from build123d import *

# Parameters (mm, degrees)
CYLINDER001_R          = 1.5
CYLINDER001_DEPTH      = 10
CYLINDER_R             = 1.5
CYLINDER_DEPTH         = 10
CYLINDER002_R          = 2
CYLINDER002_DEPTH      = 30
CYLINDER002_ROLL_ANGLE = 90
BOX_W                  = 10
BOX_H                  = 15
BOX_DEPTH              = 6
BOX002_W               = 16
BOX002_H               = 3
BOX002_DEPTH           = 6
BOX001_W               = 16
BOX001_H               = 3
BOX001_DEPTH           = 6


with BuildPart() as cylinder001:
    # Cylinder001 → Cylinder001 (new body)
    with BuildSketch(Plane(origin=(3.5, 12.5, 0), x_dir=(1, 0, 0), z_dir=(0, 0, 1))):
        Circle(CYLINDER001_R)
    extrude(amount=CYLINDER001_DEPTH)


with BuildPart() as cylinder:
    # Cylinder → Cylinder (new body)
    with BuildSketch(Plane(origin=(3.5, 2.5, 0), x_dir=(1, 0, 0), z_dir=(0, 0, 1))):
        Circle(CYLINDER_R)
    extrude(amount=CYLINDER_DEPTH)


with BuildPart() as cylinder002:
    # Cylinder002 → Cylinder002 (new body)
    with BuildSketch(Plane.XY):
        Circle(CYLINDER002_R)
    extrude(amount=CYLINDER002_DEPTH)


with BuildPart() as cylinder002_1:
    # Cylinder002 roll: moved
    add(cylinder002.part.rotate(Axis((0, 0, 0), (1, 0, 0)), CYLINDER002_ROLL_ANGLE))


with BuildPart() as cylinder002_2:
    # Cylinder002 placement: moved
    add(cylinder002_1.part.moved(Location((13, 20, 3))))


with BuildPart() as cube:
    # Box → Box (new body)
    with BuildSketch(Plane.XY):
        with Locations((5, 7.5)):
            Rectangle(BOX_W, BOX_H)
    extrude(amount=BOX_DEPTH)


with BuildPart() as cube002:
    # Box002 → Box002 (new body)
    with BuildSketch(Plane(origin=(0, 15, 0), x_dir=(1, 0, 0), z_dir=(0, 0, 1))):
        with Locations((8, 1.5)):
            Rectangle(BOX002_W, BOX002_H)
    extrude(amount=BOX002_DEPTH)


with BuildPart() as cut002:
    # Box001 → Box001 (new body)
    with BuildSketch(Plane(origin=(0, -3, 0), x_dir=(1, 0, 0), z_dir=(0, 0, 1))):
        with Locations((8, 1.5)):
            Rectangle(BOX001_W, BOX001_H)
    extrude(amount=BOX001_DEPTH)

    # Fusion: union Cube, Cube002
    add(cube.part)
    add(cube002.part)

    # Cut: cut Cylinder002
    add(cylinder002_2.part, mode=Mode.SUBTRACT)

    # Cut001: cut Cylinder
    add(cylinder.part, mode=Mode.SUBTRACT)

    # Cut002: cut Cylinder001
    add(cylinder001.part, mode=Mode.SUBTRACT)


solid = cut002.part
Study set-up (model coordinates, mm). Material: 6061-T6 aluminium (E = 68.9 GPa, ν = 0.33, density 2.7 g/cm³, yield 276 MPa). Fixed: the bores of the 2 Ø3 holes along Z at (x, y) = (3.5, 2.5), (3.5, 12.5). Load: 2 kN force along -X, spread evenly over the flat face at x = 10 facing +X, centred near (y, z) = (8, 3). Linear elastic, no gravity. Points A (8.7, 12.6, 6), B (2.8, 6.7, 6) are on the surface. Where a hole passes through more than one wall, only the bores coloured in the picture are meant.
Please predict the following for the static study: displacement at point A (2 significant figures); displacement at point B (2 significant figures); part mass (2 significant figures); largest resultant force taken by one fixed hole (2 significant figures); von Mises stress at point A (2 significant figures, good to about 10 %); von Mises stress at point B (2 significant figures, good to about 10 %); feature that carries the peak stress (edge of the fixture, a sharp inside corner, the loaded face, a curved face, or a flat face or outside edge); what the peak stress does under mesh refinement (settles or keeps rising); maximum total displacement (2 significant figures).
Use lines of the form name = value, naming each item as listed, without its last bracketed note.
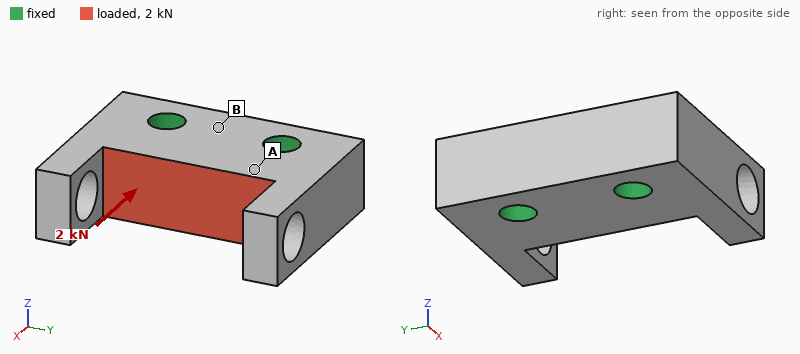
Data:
displacement at point A = 1.5 µm
displacement at point B = 0.95 µm
part mass = 3.6 g
largest resultant force taken by one fixed hole = 1.0 kN
von Mises stress at point A = 22 MPa
von Mises stress at point B = 7.3 MPa
feature that carries the peak stress = edge of the fixture
what the peak stress does under mesh refinement = keeps rising
maximum total displacement = 2.4 µm
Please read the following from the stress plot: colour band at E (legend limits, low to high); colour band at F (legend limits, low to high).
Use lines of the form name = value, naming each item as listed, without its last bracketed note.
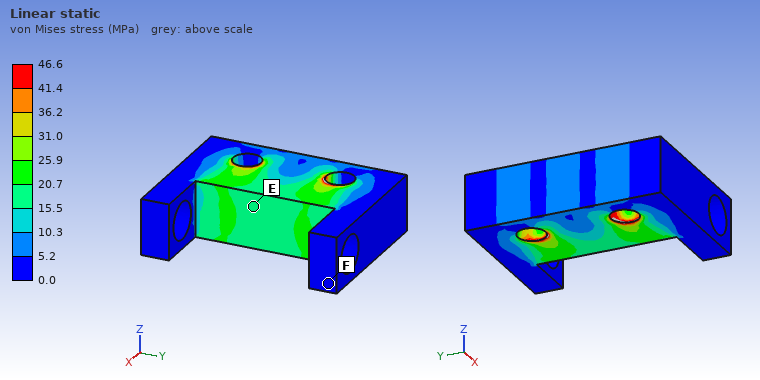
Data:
colour band at E = 15.5 to 20.7 MPa
colour band at F = 0.0 to 5.2 MPa
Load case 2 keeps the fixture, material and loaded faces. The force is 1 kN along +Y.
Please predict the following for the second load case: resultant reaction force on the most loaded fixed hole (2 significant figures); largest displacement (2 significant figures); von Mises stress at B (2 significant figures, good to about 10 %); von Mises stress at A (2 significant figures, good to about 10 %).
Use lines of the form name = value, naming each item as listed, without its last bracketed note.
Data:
resultant reaction force on the most loaded fixed hole = 670 N
largest displacement = 5.5 µm
von Mises stress at B = 4.1 MPa
von Mises stress at A = 14 MPa
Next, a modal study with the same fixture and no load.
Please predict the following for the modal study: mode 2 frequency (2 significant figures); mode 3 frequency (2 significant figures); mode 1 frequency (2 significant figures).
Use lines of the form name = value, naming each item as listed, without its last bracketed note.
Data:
mode 2 frequency = 34 kHz
mode 3 frequency = 35 kHz
mode 1 frequency = 34 kHz
